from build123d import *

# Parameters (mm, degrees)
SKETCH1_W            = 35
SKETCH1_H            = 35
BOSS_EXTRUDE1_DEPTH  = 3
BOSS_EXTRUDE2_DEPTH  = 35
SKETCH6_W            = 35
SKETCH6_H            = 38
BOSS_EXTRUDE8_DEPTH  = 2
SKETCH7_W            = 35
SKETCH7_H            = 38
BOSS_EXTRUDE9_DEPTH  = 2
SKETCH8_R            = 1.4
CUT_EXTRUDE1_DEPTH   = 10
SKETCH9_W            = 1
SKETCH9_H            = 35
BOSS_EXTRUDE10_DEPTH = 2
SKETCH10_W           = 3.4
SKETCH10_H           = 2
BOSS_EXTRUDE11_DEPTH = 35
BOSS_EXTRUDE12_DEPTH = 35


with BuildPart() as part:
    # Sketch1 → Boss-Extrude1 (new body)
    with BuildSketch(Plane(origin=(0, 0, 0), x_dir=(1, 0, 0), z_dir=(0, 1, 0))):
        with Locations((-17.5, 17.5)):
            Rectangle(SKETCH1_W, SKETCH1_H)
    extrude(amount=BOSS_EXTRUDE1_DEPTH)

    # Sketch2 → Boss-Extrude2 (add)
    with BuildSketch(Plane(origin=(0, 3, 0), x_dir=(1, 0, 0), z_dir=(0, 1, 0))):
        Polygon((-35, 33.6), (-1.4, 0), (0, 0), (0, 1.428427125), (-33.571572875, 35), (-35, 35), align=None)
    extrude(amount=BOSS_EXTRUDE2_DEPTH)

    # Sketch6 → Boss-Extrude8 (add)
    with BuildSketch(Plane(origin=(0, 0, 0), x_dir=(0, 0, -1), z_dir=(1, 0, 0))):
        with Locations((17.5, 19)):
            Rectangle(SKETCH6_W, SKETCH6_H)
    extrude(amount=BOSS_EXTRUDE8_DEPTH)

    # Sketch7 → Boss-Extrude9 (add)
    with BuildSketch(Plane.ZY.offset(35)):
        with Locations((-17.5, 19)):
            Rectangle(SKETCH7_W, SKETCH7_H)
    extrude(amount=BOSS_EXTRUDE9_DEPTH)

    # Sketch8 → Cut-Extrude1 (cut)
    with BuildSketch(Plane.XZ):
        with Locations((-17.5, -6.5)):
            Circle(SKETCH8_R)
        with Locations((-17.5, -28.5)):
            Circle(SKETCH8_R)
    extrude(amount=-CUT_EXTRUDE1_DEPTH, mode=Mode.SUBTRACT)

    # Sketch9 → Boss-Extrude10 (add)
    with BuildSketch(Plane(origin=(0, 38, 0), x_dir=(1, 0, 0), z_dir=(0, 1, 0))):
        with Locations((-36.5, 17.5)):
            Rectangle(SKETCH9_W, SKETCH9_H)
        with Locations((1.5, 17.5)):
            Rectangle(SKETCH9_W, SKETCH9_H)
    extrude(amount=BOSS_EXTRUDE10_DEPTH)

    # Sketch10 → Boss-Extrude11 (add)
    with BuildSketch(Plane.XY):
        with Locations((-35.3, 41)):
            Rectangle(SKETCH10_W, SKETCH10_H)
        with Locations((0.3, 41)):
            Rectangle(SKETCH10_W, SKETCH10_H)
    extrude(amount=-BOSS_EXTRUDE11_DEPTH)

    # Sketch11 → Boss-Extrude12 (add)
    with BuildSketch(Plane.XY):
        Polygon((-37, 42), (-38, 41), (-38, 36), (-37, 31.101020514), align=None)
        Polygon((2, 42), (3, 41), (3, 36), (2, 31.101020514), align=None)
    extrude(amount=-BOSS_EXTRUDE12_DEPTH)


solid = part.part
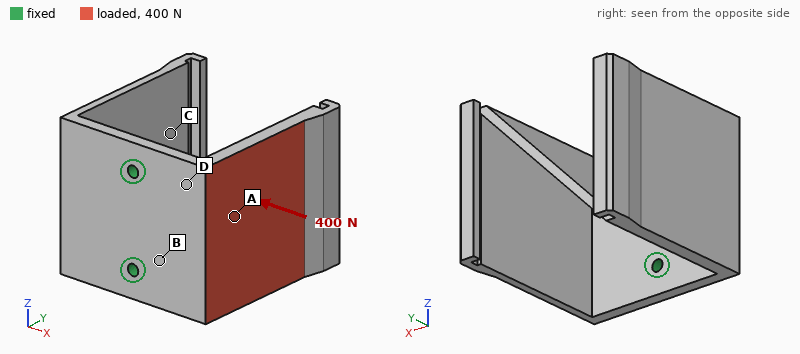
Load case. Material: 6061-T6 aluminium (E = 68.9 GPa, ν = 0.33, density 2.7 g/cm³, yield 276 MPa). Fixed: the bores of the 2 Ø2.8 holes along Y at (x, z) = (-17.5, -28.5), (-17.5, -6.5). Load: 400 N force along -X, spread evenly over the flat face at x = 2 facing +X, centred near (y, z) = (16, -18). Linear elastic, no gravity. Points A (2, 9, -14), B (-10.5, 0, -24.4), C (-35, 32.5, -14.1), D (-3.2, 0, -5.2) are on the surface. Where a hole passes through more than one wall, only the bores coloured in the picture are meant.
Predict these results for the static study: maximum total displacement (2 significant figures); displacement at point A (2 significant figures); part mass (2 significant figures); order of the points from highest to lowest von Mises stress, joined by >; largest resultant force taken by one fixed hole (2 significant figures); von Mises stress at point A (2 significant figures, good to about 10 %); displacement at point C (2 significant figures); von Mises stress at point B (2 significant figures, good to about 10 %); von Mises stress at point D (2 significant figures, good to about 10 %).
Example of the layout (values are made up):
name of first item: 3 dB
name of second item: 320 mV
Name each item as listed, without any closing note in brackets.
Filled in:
maximum total displacement: 0.66 mm
displacement at point A: 0.12 mm
part mass: 37 g
order of the points from highest to lowest von Mises stress, joined by >: B > A > D > C
largest resultant force taken by one fixed hole: 200 N
von Mises stress at point A: 39 MPa
displacement at point C: 0.13 mm
von Mises stress at point B: 50 MPa
von Mises stress at point D: 19 MPa
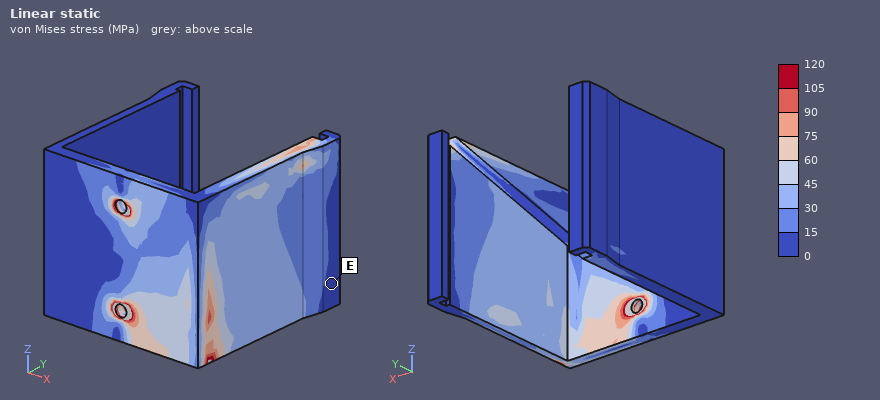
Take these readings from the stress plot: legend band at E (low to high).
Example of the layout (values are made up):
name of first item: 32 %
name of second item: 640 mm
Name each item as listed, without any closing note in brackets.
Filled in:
legend band at E: 0 to 15 MPa
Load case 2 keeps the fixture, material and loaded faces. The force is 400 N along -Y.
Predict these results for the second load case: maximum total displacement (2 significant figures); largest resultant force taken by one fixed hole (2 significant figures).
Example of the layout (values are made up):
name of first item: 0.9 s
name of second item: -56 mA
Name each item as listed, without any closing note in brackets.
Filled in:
maximum total displacement: 0.40 mm
largest resultant force taken by one fixed hole: 210 N
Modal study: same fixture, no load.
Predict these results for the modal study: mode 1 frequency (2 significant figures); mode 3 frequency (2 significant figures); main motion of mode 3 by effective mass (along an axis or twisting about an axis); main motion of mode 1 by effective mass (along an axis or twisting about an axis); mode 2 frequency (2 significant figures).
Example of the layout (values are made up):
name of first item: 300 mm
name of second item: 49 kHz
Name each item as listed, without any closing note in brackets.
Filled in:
mode 1 frequency: 1100 Hz
mode 3 frequency: 2600 Hz
main motion of mode 3 by effective mass: along Z
main motion of mode 1 by effective mass: along X
mode 2 frequency: 1500 Hz
